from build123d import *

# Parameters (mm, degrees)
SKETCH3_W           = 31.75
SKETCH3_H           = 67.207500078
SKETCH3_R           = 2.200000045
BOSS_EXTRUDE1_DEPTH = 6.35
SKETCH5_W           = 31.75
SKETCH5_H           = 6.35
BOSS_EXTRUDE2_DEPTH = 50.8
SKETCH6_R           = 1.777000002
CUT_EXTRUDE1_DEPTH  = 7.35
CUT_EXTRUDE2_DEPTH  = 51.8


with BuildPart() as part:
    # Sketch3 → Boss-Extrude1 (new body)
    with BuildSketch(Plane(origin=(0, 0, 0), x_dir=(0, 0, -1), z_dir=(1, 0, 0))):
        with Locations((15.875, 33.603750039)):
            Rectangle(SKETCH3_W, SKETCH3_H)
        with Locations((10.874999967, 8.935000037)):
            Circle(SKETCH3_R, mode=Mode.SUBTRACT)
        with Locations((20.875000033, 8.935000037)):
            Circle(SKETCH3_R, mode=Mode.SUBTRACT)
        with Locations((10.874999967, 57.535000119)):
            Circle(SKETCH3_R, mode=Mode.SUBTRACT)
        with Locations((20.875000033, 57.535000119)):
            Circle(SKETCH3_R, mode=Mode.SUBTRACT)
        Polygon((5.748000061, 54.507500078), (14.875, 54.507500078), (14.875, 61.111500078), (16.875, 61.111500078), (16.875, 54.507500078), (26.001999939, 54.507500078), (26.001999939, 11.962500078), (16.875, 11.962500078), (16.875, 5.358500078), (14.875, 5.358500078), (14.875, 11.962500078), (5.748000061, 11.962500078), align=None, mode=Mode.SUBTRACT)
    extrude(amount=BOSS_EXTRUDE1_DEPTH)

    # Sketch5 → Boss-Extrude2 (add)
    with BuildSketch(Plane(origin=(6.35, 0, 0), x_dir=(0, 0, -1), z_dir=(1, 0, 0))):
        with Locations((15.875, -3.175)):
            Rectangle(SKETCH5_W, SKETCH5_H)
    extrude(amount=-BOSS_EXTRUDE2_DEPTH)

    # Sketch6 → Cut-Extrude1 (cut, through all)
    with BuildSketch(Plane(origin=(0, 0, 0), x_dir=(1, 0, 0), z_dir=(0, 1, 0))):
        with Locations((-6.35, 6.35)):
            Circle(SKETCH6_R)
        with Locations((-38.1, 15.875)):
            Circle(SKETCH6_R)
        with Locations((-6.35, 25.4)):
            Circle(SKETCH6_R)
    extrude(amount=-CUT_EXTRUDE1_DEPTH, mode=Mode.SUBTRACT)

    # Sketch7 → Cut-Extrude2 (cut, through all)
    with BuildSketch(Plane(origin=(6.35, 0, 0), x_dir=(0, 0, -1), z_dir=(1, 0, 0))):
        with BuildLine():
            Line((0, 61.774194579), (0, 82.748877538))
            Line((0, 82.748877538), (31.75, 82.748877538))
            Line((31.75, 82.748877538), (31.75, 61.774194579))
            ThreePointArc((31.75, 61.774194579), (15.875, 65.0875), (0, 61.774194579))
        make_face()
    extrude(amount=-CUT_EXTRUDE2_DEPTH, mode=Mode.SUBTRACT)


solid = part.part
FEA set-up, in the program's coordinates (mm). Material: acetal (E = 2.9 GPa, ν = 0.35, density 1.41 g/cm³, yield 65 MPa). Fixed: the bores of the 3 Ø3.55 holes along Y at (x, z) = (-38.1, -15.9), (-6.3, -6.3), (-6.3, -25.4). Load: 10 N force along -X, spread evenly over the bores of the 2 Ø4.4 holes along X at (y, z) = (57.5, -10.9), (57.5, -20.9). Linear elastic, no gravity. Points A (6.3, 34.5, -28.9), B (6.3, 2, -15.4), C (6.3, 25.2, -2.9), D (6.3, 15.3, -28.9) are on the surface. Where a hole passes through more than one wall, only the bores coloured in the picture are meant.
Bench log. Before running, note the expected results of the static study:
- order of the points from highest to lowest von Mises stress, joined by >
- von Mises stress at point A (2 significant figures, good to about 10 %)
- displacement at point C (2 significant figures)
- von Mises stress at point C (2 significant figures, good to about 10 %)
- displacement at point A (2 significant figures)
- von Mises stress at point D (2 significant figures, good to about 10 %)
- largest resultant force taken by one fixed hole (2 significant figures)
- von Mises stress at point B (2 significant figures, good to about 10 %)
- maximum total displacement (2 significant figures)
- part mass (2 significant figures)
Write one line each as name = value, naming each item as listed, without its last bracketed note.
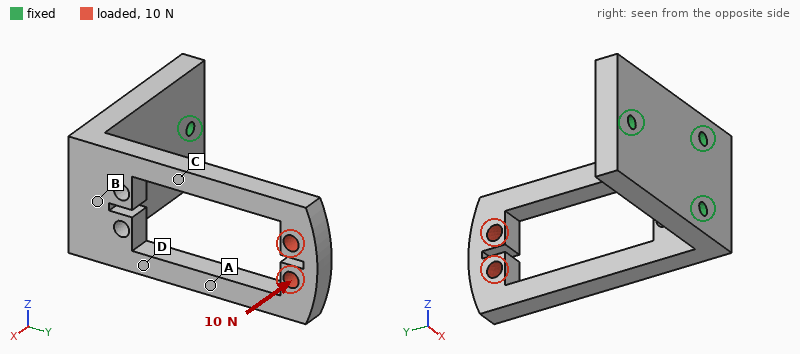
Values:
order of the points from highest to lowest von Mises stress, joined by > = D > C > A > B
von Mises stress at point A = 3.0 MPa
displacement at point C = 0.25 mm
von Mises stress at point C = 4.2 MPa
displacement at point A = 0.41 mm
von Mises stress at point D = 5.5 MPa
largest resultant force taken by one fixed hole = 5.6 N
von Mises stress at point B = 1.6 MPa
maximum total displacement = 1.1 mm
part mass = 24 g
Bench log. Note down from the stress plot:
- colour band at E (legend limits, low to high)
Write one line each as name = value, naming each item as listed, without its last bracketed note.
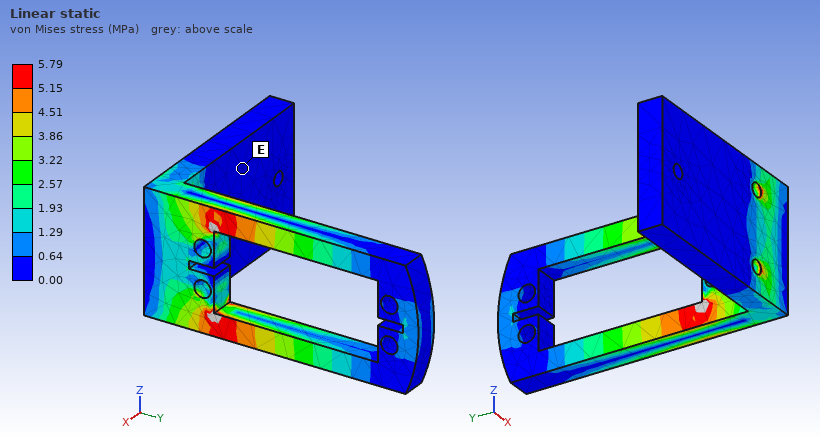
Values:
colour band at E = 0.00 to 0.64 MPa
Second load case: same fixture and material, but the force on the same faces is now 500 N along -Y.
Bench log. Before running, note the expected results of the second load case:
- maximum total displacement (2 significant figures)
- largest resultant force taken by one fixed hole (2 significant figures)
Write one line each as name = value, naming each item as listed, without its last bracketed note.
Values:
maximum total displacement = 1.1 mm
largest resultant force taken by one fixed hole = 260 N
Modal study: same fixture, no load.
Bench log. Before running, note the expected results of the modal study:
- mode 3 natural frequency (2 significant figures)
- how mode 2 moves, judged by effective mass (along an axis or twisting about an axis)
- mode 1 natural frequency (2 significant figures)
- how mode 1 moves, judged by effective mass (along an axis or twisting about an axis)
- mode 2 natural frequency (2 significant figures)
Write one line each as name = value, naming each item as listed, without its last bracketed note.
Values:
mode 3 natural frequency = 820 Hz
how mode 2 moves, judged by effective mass = along Z
mode 1 natural frequency = 270 Hz
how mode 1 moves, judged by effective mass = along X
mode 2 natural frequency = 510 Hz
